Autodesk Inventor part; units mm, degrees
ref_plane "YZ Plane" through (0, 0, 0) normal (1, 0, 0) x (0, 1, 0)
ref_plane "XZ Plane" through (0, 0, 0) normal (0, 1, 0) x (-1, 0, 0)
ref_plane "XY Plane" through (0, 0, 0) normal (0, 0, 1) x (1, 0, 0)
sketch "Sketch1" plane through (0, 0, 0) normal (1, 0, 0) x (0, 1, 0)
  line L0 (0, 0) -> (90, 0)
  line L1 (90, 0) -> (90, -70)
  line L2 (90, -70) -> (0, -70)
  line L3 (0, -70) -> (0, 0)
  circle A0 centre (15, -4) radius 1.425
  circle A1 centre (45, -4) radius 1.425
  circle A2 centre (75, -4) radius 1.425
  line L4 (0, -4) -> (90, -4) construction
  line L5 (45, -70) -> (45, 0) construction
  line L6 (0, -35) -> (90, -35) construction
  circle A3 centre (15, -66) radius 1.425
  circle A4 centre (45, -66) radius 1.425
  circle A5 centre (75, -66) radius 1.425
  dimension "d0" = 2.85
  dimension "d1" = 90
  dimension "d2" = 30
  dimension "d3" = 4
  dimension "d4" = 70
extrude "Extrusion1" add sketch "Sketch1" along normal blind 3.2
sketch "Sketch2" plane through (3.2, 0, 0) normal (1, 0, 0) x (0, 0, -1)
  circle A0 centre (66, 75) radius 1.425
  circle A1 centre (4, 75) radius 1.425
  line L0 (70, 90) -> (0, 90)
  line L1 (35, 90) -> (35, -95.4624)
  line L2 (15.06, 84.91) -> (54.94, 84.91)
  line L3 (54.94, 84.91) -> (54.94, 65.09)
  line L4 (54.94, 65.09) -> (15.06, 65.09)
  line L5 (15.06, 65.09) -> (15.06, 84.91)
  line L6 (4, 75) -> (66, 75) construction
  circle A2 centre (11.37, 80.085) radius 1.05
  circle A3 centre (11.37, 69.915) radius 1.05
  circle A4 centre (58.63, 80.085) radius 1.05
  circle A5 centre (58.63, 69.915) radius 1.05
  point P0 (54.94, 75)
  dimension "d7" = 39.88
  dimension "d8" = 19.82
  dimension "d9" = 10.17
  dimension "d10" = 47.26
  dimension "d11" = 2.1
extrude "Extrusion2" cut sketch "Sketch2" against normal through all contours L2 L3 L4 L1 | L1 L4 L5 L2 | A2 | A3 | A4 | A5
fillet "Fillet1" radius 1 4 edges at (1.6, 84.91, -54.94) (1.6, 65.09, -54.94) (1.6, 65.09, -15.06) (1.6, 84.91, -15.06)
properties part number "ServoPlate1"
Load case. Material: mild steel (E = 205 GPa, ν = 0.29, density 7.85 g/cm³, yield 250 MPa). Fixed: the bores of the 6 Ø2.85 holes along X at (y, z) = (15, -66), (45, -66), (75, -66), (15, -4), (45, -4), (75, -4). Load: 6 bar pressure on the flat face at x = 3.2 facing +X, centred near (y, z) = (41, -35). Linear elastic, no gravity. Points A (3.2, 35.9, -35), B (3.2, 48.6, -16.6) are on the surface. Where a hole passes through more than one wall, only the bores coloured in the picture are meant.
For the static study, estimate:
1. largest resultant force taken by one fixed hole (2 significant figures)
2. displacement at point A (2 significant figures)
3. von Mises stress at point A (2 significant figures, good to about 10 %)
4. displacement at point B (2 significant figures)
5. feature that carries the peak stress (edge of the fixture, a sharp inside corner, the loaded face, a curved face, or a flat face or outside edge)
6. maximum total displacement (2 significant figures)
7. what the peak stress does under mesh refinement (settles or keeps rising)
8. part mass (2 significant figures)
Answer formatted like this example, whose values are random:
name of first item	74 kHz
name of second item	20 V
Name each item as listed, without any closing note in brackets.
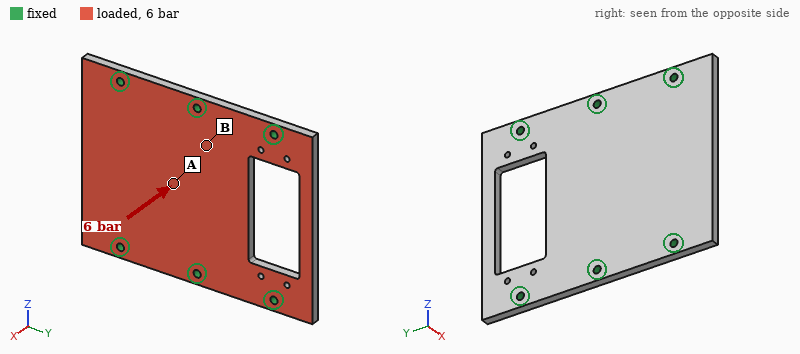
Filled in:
largest resultant force taken by one fixed hole	650 N
displacement at point A	52 µm
von Mises stress at point A	56 MPa
displacement at point B	25 µm
feature that carries the peak stress	edge of the fixture
maximum total displacement	70 µm
what the peak stress does under mesh refinement	keeps rising
part mass	140 g
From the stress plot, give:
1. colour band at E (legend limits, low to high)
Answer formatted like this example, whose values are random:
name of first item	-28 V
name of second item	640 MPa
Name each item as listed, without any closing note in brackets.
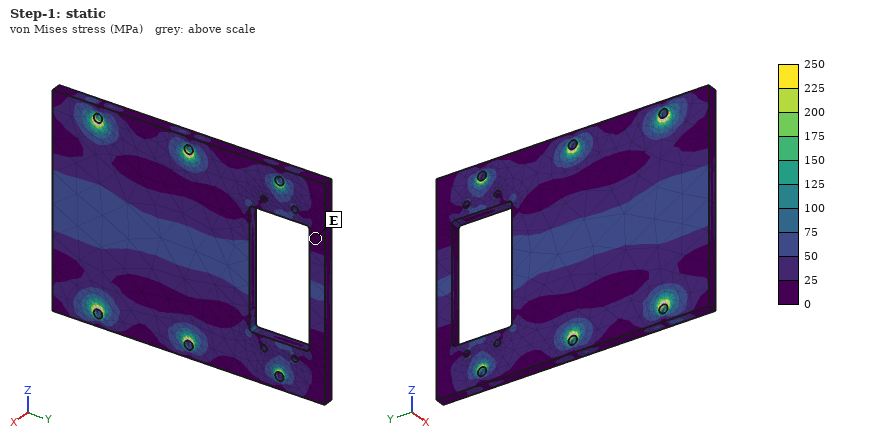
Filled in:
colour band at E	0 to 25 MPa
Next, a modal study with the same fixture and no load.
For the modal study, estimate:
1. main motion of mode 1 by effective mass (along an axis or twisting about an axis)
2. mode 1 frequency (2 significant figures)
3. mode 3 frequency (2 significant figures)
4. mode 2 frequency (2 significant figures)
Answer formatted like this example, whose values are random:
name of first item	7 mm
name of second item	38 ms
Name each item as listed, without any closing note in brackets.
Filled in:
main motion of mode 1 by effective mass	along X
mode 1 frequency	3700 Hz
mode 3 frequency	4500 Hz
mode 2 frequency	4300 Hz
